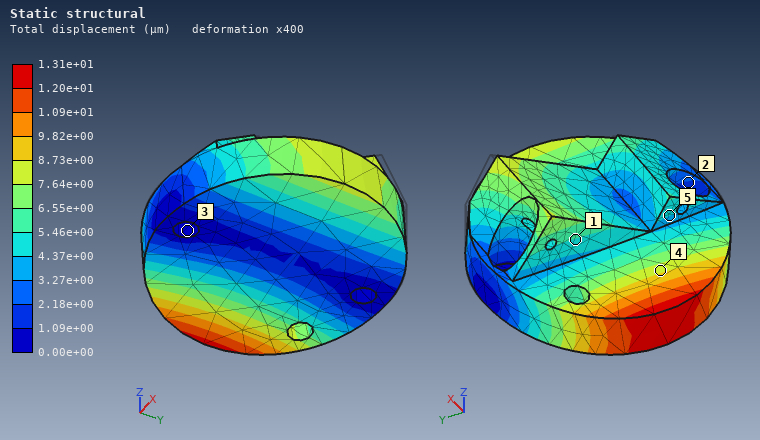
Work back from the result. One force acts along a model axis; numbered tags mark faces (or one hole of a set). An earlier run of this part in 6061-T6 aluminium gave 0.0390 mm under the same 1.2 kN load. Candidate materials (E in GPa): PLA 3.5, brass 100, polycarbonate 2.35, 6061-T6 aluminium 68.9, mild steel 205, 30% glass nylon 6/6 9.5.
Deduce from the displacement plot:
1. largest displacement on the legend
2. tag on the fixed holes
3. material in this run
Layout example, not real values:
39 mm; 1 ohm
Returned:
1.31e+01 µm; 3; mild steel
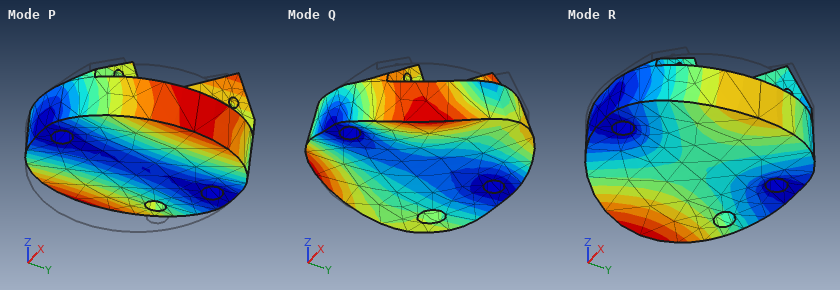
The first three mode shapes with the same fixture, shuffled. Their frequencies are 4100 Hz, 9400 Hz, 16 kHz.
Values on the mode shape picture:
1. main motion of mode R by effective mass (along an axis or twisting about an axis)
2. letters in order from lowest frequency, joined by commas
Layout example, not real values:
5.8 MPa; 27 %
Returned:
along Z; P, R, Q
